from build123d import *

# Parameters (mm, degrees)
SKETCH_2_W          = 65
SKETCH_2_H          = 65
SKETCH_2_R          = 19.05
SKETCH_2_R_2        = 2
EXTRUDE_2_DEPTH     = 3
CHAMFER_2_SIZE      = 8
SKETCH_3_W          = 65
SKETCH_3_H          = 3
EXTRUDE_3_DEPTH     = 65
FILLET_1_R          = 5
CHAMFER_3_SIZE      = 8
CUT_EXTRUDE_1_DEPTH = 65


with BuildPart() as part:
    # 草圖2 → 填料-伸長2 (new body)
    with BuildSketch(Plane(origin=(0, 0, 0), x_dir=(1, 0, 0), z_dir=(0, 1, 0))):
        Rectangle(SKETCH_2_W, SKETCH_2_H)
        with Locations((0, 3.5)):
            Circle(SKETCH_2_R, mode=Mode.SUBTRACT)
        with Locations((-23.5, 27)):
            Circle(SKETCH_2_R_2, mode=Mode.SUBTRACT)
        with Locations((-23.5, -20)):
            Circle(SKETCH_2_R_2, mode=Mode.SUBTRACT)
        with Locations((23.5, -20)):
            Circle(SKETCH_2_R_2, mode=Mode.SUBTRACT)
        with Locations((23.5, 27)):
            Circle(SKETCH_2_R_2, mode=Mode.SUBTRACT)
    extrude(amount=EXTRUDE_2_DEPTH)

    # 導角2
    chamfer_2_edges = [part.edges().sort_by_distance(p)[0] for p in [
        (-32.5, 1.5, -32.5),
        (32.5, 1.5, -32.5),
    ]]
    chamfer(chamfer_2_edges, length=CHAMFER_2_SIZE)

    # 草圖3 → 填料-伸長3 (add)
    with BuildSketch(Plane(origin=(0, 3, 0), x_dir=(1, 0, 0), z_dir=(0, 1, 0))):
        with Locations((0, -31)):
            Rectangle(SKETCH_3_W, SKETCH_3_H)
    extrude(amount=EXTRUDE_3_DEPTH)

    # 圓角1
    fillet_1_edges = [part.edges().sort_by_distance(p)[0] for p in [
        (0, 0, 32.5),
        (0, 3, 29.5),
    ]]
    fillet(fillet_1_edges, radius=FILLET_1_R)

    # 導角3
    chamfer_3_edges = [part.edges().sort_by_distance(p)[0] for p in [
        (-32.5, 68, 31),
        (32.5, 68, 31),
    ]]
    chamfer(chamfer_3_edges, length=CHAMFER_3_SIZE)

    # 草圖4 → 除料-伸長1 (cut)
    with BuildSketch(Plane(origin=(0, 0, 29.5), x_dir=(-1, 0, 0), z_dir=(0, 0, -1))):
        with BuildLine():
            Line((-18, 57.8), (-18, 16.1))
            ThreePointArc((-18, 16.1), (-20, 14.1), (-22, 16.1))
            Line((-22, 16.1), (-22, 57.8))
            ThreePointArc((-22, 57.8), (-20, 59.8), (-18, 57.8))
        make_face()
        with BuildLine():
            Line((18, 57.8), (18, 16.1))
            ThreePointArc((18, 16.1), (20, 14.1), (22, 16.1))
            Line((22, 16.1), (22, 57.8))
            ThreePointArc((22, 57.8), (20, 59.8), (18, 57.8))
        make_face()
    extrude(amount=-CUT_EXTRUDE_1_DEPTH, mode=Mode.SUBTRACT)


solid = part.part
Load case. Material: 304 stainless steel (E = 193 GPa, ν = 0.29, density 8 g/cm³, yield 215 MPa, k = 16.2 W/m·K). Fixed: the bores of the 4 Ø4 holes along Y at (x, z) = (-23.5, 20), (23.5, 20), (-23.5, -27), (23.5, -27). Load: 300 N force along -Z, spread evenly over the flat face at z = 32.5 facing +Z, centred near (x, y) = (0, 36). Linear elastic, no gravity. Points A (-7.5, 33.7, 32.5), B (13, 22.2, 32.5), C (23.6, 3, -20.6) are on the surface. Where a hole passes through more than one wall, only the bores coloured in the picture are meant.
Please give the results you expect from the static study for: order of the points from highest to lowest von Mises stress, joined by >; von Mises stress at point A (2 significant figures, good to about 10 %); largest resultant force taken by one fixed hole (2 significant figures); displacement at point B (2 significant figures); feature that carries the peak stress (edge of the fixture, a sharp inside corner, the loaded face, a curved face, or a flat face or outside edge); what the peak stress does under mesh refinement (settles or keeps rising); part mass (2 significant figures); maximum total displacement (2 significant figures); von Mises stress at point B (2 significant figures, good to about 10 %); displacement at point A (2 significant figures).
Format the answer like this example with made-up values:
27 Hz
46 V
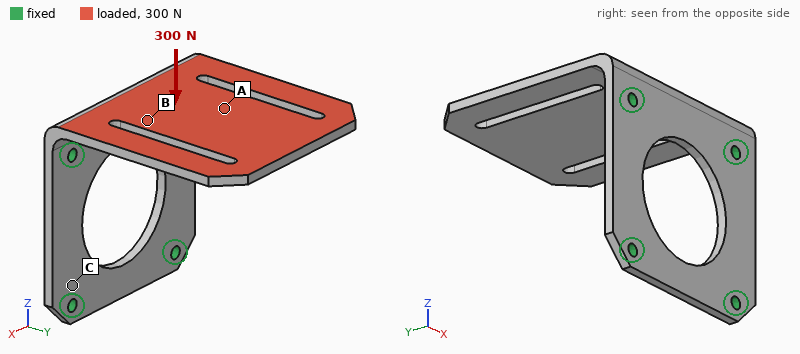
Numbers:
B > A > C
30 MPa
160 N
0.12 mm
edge of the fixture
keeps rising
160 g
0.59 mm
55 MPa
0.23 mm
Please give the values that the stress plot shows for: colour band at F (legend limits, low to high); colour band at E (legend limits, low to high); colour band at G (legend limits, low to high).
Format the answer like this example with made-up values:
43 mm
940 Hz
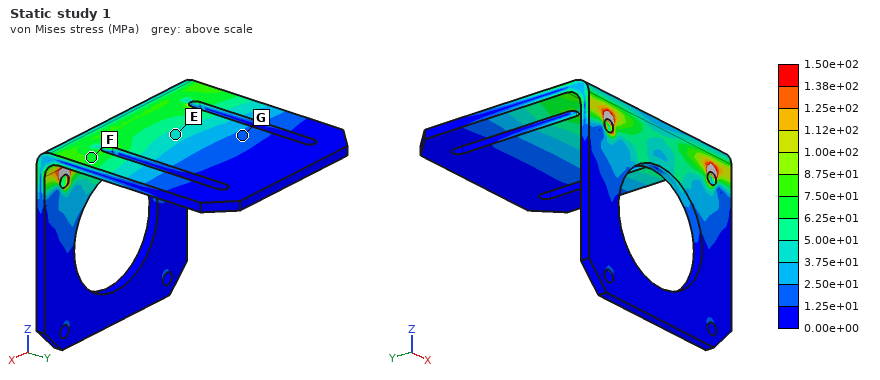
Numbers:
6.25e+01 to 7.50e+01 MPa
3.75e+01 to 5.00e+01 MPa
1.25e+01 to 2.50e+01 MPa
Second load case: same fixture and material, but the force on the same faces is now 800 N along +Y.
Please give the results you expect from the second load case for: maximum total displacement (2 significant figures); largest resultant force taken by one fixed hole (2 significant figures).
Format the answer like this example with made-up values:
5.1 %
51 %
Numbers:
0.22 mm
410 N
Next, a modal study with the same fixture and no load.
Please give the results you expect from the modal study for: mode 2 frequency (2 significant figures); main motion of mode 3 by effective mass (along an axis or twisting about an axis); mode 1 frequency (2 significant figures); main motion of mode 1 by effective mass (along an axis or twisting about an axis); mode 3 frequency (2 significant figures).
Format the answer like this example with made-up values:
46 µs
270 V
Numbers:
1300 Hz
along X
470 Hz
along Z
2500 Hz
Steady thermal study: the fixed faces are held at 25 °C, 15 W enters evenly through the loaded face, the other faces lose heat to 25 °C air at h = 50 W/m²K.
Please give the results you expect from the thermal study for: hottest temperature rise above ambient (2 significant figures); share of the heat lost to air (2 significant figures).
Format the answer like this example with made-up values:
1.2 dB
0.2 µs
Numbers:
55 K
79 %
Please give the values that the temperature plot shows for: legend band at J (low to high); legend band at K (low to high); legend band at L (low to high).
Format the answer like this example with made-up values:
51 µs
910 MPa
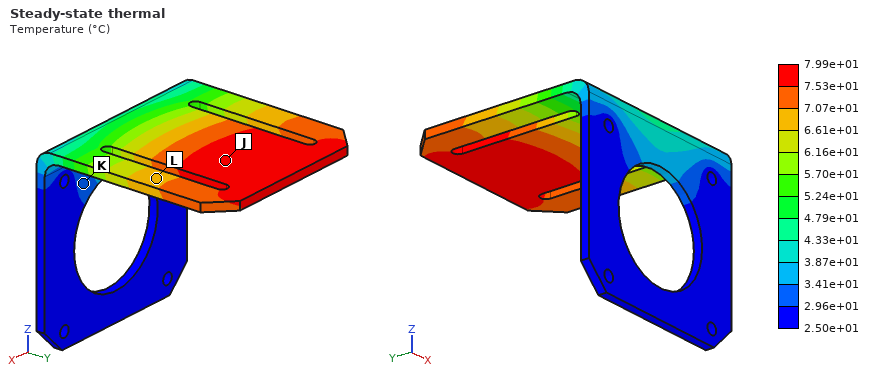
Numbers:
7.53e+01 to 7.99e+01 °C
2.96e+01 to 3.41e+01 °C
6.61e+01 to 7.07e+01 °C
